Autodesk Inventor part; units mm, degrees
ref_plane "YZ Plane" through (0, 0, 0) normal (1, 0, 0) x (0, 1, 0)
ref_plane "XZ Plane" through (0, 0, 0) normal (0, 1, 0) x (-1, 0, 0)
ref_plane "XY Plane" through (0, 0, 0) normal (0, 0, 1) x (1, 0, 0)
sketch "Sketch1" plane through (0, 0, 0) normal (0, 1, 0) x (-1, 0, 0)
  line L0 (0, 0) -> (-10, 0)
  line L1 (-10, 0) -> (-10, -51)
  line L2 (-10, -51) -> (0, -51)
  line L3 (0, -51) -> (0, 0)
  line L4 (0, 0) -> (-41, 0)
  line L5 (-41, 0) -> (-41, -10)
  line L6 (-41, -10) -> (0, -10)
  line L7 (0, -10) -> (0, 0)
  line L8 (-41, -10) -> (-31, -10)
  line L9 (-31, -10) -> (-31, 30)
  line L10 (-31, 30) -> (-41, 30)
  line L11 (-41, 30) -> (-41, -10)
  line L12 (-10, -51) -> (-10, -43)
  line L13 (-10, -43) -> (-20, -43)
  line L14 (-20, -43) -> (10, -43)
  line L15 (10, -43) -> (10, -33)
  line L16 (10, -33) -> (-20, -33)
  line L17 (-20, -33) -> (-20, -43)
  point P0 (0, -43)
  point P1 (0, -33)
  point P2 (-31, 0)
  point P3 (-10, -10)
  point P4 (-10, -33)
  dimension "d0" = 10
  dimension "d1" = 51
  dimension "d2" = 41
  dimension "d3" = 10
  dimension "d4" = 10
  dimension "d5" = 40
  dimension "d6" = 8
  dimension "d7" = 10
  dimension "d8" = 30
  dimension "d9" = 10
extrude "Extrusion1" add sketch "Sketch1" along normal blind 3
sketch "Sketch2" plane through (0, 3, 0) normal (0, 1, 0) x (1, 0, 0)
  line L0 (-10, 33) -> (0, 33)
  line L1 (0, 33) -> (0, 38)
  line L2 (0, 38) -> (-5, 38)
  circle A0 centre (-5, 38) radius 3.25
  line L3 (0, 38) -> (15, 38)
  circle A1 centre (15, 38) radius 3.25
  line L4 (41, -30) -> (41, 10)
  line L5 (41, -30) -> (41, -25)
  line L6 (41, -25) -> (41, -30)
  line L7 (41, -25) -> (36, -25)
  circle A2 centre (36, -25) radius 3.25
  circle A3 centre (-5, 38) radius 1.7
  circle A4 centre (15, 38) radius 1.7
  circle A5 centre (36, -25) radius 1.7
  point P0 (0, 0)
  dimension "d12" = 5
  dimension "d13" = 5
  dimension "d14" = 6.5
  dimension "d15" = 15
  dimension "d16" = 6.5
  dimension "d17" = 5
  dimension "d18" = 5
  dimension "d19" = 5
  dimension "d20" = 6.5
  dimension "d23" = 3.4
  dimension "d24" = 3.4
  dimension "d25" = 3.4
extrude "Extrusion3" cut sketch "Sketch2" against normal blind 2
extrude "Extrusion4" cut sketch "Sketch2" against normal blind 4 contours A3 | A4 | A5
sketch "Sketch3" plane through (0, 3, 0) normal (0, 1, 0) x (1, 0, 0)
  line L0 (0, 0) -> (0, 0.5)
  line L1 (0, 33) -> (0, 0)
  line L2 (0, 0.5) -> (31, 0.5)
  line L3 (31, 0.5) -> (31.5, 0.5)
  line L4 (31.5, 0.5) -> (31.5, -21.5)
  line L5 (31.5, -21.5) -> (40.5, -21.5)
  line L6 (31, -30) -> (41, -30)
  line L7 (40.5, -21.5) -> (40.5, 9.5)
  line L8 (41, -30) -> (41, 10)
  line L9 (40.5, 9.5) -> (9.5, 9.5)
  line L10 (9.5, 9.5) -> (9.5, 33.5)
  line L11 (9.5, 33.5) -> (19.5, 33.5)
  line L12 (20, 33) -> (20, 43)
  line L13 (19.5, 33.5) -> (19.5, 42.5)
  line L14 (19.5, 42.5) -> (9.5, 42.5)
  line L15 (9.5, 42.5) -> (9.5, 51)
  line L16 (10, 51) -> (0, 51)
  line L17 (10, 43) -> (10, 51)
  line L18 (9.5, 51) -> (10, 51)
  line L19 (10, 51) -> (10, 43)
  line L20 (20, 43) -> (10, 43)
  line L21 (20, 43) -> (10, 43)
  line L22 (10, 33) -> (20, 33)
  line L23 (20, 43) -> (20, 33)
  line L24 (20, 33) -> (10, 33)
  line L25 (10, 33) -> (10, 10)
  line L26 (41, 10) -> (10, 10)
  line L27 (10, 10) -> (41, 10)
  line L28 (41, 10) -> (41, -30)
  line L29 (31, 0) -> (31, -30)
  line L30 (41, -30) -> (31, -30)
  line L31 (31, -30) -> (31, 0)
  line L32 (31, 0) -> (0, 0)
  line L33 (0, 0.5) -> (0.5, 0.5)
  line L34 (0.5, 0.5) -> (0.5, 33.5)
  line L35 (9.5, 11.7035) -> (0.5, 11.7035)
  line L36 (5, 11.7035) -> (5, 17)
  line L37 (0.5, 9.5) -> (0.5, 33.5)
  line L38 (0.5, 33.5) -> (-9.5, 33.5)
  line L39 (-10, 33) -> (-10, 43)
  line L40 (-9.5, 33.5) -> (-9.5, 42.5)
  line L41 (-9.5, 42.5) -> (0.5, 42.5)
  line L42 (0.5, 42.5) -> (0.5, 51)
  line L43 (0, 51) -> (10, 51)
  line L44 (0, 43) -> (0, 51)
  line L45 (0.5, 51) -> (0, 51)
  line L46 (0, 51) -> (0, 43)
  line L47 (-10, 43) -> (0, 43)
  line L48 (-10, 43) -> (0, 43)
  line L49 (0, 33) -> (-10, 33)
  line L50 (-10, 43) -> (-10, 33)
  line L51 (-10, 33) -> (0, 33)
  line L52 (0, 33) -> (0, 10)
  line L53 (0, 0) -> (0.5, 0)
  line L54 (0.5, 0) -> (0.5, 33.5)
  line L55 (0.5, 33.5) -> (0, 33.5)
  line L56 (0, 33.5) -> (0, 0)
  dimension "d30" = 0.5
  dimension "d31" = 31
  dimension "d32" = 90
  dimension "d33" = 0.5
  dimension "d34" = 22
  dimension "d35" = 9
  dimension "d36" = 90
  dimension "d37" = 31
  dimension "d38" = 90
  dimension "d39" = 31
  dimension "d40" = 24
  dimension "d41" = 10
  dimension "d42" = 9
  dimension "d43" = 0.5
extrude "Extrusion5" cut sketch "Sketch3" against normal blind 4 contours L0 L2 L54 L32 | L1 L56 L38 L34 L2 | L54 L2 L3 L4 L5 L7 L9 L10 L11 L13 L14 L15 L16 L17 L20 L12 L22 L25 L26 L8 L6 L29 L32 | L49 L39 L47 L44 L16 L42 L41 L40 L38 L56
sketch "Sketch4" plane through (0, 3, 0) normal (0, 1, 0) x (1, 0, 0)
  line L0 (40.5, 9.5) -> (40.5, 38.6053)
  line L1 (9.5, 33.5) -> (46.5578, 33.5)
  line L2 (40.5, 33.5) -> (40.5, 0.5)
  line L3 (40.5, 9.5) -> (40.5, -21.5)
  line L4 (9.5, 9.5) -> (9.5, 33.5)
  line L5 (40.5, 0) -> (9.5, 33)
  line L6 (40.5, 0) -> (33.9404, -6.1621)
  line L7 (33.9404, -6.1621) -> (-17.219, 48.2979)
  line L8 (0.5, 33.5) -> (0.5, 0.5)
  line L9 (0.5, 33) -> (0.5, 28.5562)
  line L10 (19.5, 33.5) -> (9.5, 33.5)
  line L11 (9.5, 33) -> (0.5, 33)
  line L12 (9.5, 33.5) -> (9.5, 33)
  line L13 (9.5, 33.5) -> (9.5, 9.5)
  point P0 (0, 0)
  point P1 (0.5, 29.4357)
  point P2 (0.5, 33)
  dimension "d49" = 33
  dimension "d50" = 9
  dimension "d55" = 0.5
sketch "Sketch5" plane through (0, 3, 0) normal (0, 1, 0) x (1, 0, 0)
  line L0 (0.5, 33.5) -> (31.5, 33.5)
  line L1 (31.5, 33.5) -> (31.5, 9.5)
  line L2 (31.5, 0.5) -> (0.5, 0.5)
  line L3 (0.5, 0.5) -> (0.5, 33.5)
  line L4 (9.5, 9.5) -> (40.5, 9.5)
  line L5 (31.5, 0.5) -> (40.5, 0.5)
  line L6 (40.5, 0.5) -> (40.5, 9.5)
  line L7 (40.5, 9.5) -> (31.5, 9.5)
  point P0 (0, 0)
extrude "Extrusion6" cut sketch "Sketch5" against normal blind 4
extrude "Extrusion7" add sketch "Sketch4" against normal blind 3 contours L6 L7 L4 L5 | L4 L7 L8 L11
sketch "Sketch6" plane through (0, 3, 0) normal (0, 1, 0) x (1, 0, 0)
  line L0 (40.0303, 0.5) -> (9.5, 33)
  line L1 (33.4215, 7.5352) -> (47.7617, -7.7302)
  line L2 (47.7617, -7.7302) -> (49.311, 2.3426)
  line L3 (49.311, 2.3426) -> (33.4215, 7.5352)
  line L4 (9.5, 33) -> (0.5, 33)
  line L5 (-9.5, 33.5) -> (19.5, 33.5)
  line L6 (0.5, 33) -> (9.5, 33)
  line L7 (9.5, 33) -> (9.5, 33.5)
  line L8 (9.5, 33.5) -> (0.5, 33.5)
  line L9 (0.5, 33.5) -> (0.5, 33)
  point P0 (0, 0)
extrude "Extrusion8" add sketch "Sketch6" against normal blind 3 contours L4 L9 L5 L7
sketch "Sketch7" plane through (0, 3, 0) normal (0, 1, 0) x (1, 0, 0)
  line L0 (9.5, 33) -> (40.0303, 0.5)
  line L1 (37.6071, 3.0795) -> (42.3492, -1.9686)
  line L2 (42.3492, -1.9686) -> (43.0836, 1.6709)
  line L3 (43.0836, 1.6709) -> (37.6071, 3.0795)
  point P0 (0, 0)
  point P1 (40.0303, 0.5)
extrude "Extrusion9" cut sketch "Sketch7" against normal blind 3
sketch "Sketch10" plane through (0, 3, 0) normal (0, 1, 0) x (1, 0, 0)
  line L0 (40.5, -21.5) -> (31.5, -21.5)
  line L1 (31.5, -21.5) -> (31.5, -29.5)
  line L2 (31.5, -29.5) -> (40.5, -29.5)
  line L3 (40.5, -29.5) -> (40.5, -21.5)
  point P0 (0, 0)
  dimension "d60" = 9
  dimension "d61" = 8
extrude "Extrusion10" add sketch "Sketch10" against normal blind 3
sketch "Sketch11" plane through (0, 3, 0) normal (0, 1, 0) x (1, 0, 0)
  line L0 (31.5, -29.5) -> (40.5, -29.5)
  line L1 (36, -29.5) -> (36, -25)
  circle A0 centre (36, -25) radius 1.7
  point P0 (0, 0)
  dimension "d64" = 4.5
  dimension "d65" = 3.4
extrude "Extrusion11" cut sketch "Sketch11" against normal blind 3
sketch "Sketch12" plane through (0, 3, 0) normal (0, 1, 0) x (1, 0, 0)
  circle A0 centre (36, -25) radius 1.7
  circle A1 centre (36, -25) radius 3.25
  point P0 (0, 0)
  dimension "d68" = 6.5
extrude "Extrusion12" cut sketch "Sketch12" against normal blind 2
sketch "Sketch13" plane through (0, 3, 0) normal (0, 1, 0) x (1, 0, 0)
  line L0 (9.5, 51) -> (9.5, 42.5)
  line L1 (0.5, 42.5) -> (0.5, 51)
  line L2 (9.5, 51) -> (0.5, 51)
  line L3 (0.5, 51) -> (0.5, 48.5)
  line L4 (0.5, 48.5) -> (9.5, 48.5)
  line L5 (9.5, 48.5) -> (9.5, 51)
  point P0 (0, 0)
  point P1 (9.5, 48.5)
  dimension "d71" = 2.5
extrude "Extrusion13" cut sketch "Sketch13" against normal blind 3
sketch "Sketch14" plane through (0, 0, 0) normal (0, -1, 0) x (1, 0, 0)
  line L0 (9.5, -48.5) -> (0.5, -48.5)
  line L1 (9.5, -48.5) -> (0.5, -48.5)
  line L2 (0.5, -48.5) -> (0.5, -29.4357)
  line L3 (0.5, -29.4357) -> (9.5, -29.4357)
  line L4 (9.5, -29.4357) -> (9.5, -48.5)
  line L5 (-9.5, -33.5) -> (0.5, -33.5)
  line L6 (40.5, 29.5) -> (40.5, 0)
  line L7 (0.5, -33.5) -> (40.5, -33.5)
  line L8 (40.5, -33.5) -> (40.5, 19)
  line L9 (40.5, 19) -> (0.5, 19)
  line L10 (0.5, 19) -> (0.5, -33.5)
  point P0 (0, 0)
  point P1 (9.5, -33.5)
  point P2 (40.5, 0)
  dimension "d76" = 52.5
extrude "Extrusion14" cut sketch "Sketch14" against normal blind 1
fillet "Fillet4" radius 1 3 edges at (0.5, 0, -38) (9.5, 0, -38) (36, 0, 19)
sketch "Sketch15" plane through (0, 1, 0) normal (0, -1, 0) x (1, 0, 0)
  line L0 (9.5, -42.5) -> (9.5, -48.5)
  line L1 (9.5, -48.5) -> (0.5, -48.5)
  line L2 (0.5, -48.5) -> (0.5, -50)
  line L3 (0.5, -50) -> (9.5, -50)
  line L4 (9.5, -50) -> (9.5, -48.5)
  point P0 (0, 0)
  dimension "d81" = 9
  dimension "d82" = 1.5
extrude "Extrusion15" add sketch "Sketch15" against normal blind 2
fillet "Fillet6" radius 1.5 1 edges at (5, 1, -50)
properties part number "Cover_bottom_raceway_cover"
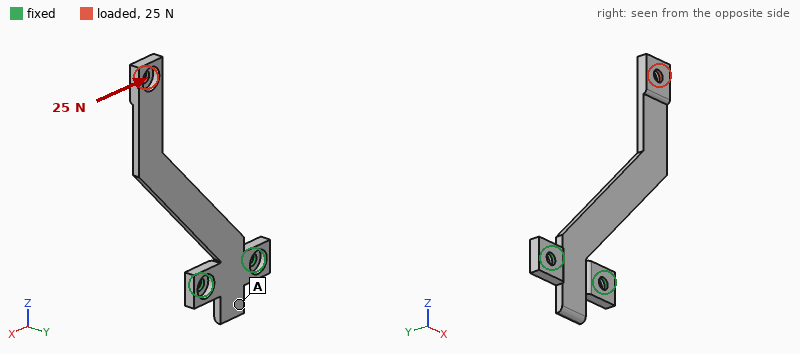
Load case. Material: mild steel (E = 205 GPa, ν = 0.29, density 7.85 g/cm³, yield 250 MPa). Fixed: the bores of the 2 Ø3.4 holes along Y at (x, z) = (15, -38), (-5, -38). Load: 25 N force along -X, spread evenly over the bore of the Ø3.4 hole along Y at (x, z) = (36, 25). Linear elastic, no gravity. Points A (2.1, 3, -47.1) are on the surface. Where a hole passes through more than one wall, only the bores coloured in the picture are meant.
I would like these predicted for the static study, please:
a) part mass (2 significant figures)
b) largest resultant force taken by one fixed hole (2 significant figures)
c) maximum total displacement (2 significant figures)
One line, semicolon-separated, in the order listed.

16 g; 87 N; 0.13 mm
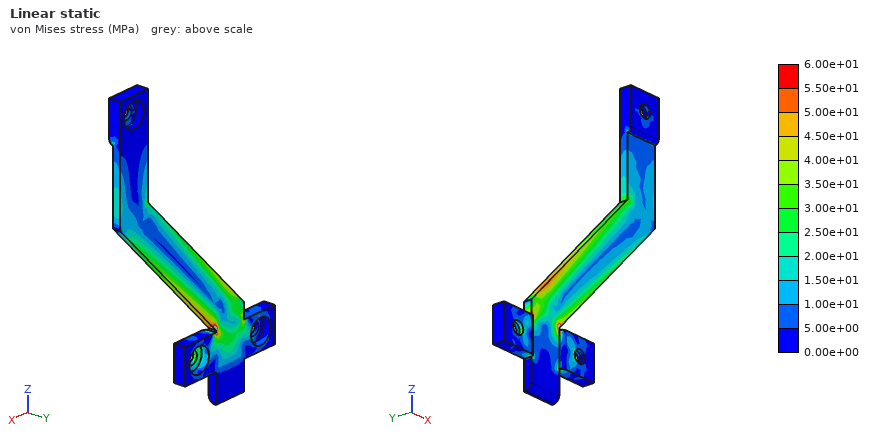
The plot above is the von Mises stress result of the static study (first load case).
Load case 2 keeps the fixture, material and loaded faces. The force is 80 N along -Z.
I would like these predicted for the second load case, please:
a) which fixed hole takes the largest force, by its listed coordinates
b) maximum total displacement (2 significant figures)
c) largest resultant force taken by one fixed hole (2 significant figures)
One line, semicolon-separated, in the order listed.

(15, -38); 0.29 mm; 180 N
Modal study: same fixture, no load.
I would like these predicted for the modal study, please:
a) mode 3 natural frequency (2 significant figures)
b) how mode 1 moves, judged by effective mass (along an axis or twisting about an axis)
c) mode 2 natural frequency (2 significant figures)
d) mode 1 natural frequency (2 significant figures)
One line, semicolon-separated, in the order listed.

1600 Hz; along Y; 1200 Hz; 280 Hz
